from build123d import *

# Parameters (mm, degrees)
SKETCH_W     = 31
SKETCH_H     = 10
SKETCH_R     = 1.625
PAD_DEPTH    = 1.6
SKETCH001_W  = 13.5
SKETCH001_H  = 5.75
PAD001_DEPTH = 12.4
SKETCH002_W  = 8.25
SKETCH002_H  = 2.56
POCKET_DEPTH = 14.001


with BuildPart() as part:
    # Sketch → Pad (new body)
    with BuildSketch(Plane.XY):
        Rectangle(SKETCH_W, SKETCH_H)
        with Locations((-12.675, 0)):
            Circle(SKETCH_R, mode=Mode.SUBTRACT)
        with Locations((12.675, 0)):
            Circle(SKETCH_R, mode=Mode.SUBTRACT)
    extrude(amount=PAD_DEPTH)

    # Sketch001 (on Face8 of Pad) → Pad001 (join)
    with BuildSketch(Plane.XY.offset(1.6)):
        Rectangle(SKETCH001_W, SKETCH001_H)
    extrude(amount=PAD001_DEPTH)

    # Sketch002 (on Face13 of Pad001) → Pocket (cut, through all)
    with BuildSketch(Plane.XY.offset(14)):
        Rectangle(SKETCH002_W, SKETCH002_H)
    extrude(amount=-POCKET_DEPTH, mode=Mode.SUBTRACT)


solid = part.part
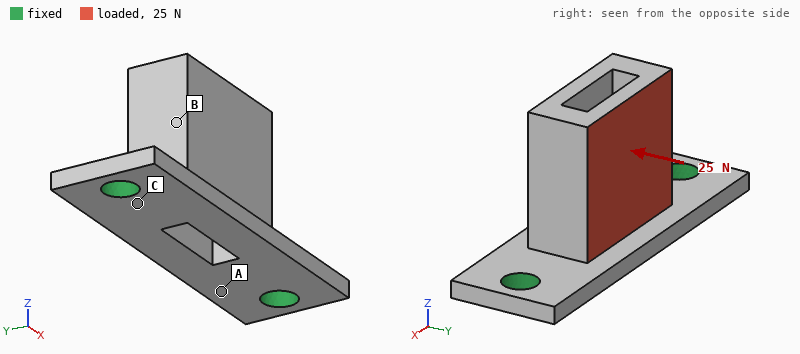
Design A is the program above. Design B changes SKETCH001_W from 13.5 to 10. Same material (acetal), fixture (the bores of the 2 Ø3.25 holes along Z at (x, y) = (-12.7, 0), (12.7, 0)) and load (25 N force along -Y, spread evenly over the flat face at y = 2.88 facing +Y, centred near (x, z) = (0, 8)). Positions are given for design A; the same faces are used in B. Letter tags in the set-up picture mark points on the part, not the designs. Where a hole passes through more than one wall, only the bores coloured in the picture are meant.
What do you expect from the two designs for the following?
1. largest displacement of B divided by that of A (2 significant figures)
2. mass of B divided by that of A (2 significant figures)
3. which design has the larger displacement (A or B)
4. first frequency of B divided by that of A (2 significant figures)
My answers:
1.4
0.78
B
1.0
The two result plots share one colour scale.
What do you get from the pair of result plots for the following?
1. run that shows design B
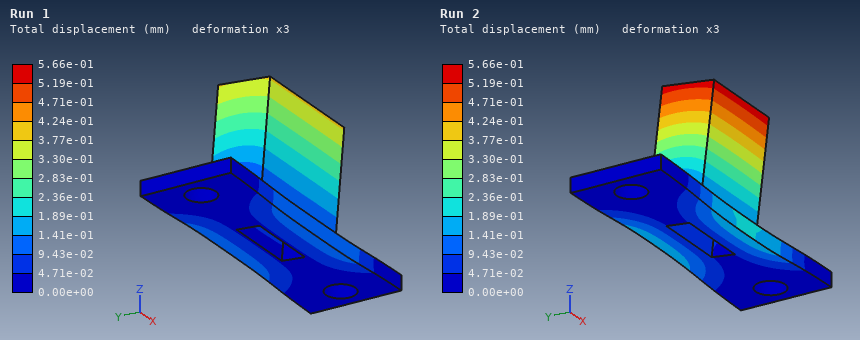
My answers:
Run 2
